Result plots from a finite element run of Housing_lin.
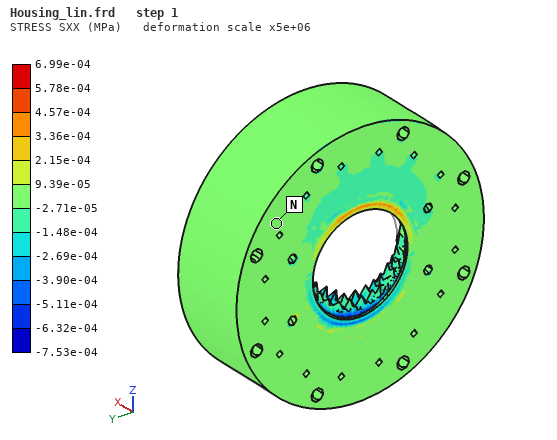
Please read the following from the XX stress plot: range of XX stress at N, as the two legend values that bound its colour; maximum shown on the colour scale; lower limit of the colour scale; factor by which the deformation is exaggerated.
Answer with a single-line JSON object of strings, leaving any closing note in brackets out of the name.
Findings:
{"range of XX stress at N, as the two legend values that bound its colour": "-2.71e-05 to 9.39e-05 MPa", "maximum shown on the colour scale": "6.99e-04 MPa", "lower limit of the colour scale": "-7.53e-04 MPa", "factor by which the deformation is exaggerated": "5e+06"}
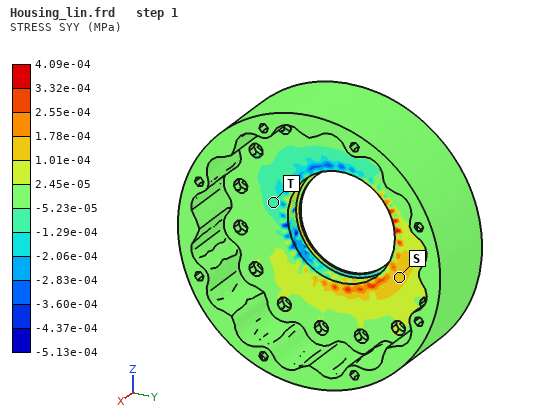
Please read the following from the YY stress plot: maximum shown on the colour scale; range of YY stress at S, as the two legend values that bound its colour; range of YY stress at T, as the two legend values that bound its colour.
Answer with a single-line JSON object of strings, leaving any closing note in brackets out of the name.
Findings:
{"maximum shown on the colour scale": "4.09e-04 MPa", "range of YY stress at S, as the two legend values that bound its colour": "1.01e-04 to 1.78e-04 MPa", "range of YY stress at T, as the two legend values that bound its colour": "-1.29e-04 to -5.23e-05 MPa"}
